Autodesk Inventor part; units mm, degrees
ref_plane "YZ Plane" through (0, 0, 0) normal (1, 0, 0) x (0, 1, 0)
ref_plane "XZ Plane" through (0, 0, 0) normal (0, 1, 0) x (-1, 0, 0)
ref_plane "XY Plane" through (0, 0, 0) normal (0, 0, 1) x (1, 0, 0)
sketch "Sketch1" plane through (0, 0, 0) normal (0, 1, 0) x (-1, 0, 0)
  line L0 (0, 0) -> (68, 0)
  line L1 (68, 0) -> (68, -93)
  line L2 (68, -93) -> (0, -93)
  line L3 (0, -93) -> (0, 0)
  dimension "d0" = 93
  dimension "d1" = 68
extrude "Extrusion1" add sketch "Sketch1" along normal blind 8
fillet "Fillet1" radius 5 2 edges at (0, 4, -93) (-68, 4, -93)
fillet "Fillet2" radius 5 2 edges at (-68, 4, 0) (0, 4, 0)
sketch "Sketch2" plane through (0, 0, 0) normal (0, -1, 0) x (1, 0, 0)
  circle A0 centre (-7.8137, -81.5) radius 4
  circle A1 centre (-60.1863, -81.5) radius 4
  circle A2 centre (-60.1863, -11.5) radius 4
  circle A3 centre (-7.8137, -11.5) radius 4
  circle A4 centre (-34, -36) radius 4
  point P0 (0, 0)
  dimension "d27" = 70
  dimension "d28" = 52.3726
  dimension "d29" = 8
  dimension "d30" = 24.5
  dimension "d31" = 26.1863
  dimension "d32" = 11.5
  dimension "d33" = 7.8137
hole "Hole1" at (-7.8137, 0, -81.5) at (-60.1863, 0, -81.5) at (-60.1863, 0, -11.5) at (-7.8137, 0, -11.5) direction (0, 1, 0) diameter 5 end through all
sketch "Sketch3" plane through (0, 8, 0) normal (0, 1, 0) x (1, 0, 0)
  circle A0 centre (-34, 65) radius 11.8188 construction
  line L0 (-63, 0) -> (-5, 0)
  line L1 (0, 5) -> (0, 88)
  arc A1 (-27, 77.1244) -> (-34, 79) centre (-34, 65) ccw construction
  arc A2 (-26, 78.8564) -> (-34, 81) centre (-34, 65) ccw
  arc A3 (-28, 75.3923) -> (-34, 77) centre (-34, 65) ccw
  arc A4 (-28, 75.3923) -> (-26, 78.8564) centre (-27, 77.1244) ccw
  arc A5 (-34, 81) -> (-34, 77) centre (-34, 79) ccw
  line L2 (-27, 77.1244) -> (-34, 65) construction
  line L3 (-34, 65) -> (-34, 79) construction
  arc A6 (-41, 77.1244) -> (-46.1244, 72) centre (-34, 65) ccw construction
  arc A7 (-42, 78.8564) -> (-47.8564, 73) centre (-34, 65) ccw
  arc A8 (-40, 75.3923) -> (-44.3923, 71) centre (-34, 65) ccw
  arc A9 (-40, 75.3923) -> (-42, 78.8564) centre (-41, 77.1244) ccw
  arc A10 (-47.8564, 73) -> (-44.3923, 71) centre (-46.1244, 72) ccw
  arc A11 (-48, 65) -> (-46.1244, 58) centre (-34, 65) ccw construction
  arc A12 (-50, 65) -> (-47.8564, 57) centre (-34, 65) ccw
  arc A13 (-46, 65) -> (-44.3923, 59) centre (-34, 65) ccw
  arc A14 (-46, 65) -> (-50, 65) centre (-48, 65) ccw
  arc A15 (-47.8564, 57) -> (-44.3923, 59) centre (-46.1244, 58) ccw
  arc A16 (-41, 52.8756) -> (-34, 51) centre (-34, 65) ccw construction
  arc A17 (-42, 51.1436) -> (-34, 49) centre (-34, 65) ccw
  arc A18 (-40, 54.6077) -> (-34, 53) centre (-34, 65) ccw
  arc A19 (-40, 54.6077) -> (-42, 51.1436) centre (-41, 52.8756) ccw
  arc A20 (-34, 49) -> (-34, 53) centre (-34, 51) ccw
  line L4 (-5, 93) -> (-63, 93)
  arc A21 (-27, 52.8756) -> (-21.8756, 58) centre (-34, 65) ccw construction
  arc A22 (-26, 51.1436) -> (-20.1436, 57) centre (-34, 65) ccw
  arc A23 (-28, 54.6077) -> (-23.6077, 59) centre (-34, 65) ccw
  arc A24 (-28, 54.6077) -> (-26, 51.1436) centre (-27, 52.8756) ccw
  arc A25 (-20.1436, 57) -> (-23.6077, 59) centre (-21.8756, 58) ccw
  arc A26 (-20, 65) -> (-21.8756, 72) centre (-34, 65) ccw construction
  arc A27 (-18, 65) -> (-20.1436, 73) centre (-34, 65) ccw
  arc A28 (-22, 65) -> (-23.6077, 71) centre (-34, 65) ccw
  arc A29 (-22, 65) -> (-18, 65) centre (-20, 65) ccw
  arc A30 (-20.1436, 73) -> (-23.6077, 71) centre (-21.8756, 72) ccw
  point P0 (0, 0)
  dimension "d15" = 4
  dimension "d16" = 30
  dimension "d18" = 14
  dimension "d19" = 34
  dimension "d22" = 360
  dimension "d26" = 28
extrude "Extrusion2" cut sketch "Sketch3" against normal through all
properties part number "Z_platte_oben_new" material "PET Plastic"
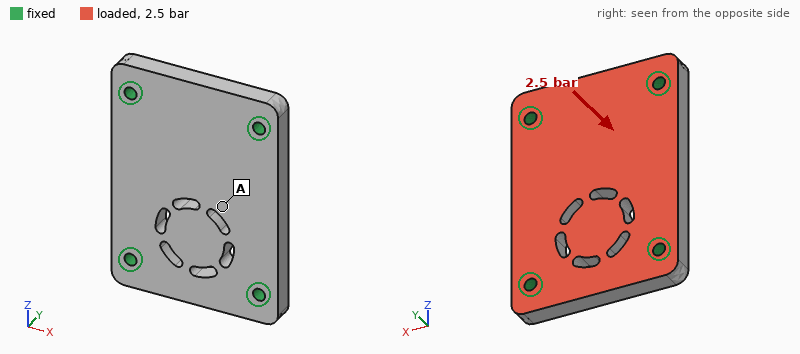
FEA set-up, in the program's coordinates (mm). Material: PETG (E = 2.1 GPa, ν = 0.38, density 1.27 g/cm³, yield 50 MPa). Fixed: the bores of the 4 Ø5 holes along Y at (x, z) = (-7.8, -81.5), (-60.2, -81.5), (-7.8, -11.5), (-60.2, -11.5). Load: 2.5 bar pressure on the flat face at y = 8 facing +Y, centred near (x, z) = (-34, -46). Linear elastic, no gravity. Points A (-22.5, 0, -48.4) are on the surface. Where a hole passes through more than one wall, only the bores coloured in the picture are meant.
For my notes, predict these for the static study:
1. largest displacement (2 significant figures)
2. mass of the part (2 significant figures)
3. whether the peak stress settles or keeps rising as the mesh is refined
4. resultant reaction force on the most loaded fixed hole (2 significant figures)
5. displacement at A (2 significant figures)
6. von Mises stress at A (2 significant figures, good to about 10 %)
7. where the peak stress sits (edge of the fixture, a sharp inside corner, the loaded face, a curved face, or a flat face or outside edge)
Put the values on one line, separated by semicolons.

0.34 mm; 61 g; keeps rising; 380 N; 0.31 mm; 4.7 MPa; edge of the fixture
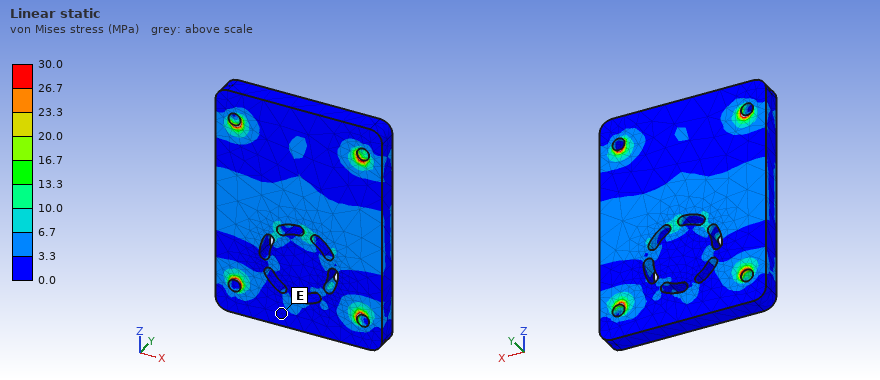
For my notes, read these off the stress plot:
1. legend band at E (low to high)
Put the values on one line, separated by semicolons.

0.0 to 3.3 MPa
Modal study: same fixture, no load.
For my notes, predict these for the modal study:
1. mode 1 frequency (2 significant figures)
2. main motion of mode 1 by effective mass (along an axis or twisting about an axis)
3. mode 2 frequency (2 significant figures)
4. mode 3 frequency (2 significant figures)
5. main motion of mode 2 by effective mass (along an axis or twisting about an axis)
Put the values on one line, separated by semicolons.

1600 Hz; along Y; 2300 Hz; 3000 Hz; twisting about Z
